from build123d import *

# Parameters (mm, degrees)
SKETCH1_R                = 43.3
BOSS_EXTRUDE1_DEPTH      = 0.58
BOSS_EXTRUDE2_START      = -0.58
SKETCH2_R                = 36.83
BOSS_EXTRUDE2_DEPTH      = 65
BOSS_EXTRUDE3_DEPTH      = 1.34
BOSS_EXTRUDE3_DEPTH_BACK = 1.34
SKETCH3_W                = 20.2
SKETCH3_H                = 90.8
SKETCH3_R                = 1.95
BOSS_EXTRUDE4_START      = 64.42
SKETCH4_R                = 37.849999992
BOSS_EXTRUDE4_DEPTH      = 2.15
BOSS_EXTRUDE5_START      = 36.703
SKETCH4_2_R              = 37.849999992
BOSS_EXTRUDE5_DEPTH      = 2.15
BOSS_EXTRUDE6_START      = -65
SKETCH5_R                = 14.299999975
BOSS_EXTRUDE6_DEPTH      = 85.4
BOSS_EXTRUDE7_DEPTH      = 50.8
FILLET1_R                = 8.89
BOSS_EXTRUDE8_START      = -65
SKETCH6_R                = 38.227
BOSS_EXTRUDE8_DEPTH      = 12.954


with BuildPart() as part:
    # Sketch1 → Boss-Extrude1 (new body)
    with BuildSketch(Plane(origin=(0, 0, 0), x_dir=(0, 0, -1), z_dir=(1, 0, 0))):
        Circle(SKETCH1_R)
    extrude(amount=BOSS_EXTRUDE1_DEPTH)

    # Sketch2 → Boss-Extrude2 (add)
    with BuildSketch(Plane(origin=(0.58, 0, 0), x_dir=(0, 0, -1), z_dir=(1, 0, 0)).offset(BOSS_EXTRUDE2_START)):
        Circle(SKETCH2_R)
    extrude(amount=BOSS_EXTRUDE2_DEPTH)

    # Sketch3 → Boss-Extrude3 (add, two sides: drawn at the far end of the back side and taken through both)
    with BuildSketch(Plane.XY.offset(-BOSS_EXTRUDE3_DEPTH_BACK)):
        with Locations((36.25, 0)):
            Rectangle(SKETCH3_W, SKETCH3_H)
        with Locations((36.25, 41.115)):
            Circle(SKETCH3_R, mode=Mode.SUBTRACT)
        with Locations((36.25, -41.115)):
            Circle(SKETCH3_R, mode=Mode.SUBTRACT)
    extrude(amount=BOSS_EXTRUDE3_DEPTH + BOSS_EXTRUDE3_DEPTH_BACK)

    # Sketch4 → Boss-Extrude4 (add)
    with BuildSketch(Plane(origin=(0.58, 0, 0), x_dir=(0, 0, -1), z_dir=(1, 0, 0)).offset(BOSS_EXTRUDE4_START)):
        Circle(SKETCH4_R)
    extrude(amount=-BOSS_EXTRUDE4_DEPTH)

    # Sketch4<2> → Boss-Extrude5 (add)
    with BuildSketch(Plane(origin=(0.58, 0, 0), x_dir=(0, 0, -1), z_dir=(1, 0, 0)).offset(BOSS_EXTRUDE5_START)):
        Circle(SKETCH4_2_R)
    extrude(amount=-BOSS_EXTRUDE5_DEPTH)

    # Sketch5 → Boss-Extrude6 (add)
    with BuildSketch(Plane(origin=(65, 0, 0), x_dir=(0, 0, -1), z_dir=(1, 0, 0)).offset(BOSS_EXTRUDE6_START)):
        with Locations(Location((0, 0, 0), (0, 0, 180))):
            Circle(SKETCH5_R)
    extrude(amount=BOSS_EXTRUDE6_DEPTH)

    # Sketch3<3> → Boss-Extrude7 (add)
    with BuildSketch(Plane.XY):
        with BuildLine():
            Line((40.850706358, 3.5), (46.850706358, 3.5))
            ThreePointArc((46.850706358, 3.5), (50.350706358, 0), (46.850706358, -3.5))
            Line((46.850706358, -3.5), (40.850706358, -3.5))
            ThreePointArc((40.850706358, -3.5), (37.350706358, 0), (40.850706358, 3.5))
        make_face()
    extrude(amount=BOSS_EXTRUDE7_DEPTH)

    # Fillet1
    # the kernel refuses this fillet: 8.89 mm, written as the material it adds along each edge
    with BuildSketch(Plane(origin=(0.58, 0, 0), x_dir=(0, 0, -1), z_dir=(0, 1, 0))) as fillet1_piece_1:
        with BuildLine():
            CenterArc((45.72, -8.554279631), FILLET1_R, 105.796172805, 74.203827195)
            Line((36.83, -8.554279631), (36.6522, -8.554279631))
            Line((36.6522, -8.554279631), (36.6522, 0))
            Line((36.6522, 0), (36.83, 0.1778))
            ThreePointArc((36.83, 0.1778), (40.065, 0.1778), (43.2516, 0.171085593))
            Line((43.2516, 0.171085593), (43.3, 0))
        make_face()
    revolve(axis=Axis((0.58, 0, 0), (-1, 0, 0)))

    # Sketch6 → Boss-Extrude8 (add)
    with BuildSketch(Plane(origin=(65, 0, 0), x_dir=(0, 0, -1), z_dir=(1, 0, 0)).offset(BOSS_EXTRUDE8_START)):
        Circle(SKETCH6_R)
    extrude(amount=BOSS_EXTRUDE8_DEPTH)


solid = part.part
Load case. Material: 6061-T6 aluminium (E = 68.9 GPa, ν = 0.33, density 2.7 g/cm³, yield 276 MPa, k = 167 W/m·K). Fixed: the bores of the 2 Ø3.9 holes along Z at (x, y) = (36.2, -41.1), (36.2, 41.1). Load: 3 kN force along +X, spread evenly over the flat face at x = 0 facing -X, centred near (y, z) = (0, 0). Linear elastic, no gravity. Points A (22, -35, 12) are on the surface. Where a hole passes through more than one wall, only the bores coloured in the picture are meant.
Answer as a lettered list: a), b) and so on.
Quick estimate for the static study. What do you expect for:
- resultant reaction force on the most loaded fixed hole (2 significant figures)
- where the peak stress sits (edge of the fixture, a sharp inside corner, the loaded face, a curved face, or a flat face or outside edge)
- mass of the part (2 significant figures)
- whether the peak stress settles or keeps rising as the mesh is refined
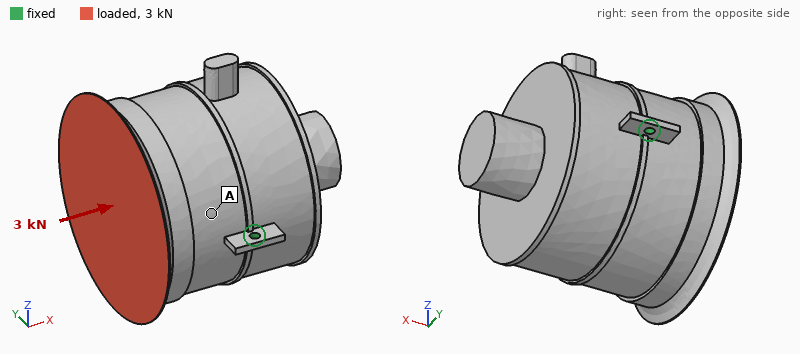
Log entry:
a) 1.5 kN
b) edge of the fixture
c) 810 g
d) keeps rising
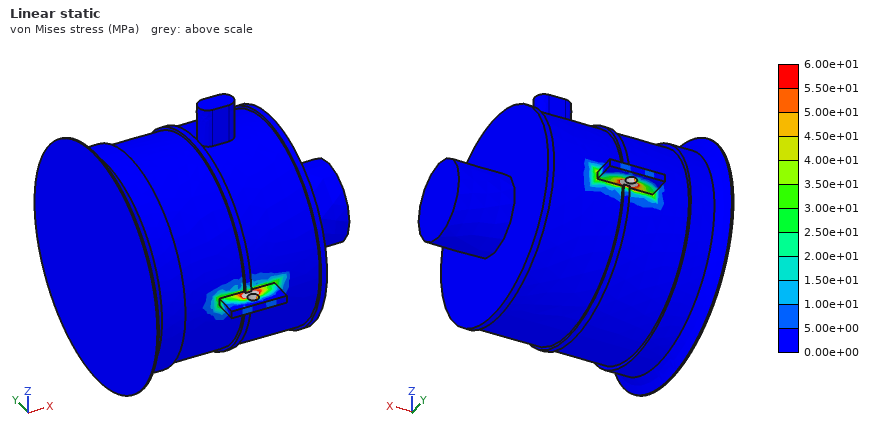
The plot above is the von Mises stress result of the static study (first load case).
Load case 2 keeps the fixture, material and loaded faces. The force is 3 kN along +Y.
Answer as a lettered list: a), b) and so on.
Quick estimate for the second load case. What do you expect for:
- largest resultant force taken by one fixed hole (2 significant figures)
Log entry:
a) 2.0 kN
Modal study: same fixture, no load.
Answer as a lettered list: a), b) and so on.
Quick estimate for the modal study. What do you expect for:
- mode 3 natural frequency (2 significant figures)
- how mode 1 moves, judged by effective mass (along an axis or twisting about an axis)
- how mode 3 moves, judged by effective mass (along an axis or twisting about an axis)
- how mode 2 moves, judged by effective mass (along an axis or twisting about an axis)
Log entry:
a) 3400 Hz
b) twisting about Y
c) along X
d) along Z
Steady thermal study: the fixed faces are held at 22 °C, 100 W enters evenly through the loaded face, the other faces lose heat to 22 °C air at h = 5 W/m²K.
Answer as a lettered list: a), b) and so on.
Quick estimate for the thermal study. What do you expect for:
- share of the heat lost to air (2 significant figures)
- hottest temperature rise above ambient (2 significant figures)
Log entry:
a) 5.0 %
b) 47 K
